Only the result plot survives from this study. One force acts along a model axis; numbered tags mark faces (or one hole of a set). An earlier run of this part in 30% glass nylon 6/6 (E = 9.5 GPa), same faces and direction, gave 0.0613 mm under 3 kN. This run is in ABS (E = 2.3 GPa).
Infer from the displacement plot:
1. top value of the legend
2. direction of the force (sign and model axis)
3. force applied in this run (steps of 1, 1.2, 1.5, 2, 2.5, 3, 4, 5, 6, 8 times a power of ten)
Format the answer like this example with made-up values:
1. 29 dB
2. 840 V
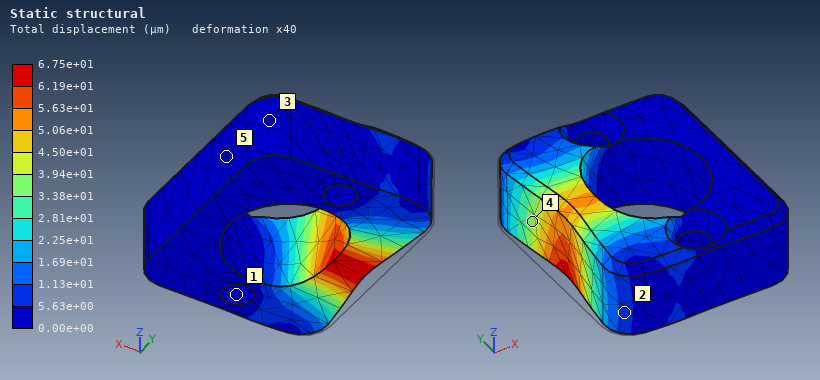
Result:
1. 6.75e+01 µm
2. +X
3. 800 N
